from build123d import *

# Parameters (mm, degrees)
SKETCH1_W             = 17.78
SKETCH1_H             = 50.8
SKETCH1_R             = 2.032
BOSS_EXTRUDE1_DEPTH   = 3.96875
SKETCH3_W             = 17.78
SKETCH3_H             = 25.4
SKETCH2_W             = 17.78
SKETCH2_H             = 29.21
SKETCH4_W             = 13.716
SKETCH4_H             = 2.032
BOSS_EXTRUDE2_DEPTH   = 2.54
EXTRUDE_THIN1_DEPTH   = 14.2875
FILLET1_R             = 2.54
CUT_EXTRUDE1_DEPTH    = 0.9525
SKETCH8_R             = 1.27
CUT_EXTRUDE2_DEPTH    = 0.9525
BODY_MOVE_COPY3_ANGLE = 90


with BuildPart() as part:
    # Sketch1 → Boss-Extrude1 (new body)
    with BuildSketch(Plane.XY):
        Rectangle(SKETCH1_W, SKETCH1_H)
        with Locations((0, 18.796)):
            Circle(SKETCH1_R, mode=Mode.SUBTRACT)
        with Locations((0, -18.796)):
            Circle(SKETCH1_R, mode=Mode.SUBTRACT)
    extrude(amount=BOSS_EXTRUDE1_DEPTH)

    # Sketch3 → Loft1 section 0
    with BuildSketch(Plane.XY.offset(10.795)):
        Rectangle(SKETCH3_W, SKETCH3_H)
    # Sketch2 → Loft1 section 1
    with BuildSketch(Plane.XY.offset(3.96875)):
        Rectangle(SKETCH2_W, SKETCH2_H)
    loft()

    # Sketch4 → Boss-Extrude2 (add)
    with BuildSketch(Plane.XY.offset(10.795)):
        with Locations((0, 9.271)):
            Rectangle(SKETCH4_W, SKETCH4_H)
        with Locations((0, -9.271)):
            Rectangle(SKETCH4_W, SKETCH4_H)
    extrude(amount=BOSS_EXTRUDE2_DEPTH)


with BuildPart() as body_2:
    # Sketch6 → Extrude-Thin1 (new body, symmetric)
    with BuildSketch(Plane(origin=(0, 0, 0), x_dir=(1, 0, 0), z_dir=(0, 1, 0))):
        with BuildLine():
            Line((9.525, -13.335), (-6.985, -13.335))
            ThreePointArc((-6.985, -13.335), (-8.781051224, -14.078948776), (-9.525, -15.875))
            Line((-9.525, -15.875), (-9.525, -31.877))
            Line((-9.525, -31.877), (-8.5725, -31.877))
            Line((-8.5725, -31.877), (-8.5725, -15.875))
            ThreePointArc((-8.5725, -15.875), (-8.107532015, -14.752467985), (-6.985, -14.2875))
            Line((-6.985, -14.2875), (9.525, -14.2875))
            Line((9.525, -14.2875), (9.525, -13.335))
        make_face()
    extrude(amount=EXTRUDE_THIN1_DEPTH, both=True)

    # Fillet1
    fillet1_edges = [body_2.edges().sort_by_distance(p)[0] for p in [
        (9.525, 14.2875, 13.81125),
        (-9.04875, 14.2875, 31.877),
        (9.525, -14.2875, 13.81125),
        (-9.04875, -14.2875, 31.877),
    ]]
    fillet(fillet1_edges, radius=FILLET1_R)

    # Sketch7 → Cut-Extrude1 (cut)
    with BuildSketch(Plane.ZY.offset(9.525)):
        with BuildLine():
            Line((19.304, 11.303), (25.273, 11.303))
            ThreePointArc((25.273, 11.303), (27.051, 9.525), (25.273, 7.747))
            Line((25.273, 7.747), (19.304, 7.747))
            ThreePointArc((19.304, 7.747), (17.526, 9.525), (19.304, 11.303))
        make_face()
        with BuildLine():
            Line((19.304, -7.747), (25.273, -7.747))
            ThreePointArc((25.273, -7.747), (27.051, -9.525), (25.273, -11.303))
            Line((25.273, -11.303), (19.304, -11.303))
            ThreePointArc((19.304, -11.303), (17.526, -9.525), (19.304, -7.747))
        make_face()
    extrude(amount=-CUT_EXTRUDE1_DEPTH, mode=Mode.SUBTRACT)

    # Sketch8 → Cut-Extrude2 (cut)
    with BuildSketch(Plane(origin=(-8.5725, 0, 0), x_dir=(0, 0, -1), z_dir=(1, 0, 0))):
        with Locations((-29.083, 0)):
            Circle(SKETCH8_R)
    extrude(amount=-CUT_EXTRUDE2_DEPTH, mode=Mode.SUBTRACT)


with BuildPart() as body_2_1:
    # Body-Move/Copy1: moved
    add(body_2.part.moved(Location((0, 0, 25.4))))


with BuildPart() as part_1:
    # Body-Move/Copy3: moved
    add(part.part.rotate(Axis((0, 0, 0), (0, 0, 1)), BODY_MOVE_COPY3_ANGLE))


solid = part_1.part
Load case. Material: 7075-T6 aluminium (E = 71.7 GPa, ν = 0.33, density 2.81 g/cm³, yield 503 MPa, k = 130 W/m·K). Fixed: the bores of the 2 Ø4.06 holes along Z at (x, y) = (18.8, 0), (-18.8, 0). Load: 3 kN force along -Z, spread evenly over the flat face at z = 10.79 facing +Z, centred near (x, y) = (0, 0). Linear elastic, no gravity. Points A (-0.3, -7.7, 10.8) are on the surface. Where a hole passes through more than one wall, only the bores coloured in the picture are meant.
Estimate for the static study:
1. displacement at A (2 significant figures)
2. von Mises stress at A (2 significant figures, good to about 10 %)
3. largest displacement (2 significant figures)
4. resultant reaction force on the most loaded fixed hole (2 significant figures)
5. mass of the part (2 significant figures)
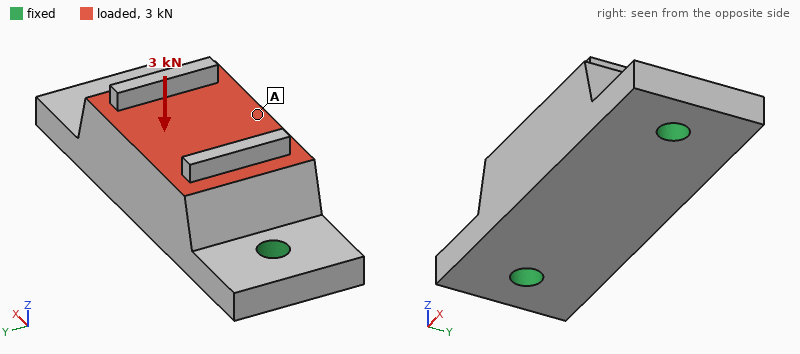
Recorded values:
20 µm
33 MPa
20 µm
1.8 kN
19 g
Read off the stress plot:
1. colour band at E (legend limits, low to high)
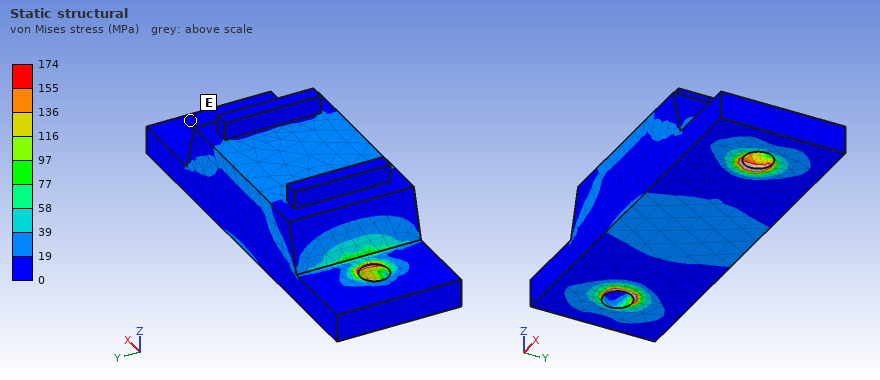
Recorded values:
0 to 19 MPa
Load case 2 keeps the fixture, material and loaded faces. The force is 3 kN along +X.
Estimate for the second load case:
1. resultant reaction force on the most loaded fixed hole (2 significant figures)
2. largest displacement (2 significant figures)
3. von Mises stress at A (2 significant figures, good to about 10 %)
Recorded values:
1.7 kN
8.7 µm
13 MPa
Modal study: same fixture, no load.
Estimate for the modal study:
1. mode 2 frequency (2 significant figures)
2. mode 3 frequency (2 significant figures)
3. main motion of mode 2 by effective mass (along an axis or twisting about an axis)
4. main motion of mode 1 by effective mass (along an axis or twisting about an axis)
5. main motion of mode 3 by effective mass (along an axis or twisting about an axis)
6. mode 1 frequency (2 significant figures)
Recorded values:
17 kHz
25 kHz
along Z
along Y
along Y
11 kHz
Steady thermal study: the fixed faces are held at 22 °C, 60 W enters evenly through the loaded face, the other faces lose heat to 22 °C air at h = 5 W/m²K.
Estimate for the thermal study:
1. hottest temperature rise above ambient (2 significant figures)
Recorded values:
37 K
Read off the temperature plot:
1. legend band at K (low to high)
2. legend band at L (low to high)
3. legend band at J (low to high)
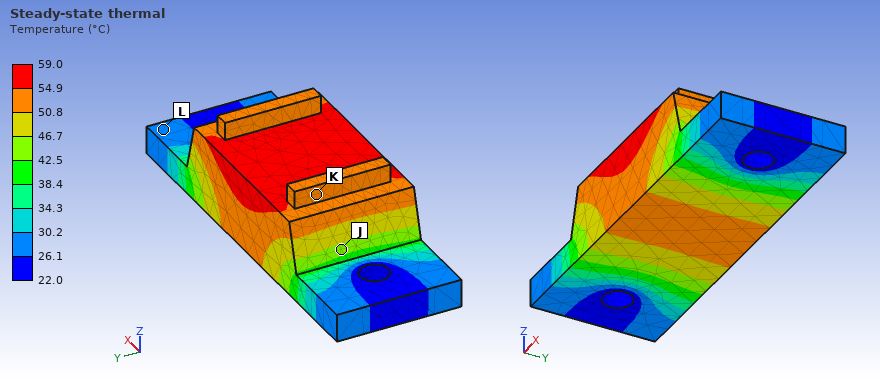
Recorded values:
50.8 to 54.9 °C
26.1 to 30.2 °C
42.5 to 46.7 °C
